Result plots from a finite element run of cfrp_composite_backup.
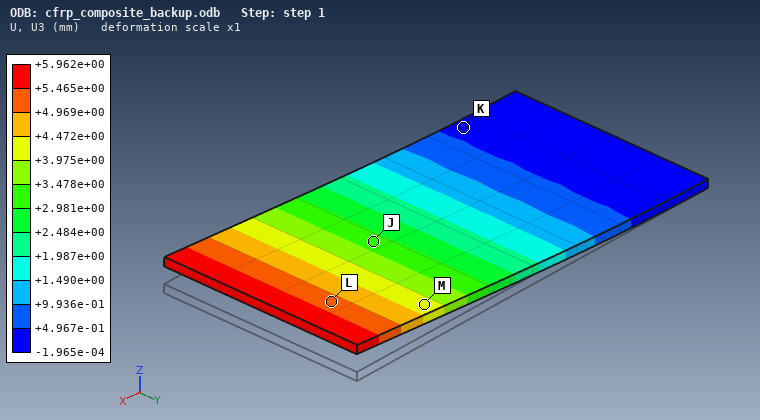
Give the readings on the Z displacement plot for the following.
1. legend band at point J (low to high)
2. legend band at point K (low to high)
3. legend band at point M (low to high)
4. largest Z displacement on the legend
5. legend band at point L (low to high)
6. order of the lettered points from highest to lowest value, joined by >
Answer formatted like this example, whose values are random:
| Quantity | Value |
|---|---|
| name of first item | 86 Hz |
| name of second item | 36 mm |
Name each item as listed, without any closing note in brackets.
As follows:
| Quantity | Value |
|---|---|
| legend band at point J | +2.981e+00 to +3.478e+00 mm |
| legend band at point K | -1.965e-04 to +4.967e-01 mm |
| legend band at point M | +3.975e+00 to +4.472e+00 mm |
| largest Z displacement on the legend | +5.962e+00 mm |
| legend band at point L | +4.969e+00 to +5.465e+00 mm |
| order of the lettered points from highest to lowest value, joined by > | L > M > J > K |
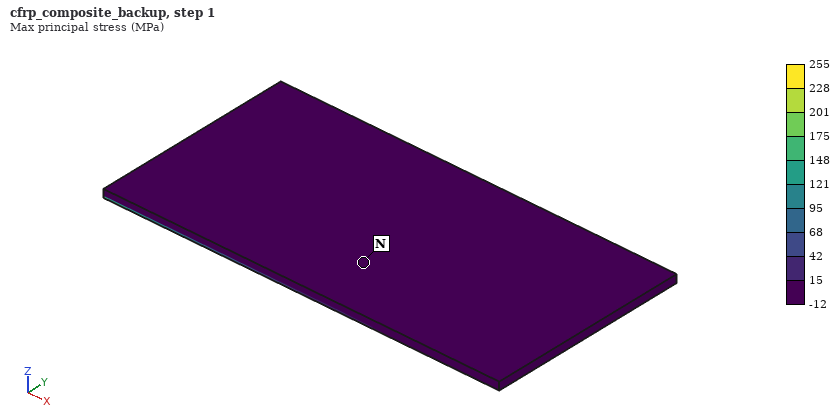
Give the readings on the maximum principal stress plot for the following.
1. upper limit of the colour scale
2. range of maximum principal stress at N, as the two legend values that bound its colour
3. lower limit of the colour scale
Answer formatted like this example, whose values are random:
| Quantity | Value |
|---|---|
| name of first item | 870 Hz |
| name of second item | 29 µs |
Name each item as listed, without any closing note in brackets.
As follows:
| Quantity | Value |
|---|---|
| upper limit of the colour scale | 255 MPa |
| range of maximum principal stress at N, as the two legend values that bound its colour | -12 to 15 MPa |
| lower limit of the colour scale | -12 MPa |
